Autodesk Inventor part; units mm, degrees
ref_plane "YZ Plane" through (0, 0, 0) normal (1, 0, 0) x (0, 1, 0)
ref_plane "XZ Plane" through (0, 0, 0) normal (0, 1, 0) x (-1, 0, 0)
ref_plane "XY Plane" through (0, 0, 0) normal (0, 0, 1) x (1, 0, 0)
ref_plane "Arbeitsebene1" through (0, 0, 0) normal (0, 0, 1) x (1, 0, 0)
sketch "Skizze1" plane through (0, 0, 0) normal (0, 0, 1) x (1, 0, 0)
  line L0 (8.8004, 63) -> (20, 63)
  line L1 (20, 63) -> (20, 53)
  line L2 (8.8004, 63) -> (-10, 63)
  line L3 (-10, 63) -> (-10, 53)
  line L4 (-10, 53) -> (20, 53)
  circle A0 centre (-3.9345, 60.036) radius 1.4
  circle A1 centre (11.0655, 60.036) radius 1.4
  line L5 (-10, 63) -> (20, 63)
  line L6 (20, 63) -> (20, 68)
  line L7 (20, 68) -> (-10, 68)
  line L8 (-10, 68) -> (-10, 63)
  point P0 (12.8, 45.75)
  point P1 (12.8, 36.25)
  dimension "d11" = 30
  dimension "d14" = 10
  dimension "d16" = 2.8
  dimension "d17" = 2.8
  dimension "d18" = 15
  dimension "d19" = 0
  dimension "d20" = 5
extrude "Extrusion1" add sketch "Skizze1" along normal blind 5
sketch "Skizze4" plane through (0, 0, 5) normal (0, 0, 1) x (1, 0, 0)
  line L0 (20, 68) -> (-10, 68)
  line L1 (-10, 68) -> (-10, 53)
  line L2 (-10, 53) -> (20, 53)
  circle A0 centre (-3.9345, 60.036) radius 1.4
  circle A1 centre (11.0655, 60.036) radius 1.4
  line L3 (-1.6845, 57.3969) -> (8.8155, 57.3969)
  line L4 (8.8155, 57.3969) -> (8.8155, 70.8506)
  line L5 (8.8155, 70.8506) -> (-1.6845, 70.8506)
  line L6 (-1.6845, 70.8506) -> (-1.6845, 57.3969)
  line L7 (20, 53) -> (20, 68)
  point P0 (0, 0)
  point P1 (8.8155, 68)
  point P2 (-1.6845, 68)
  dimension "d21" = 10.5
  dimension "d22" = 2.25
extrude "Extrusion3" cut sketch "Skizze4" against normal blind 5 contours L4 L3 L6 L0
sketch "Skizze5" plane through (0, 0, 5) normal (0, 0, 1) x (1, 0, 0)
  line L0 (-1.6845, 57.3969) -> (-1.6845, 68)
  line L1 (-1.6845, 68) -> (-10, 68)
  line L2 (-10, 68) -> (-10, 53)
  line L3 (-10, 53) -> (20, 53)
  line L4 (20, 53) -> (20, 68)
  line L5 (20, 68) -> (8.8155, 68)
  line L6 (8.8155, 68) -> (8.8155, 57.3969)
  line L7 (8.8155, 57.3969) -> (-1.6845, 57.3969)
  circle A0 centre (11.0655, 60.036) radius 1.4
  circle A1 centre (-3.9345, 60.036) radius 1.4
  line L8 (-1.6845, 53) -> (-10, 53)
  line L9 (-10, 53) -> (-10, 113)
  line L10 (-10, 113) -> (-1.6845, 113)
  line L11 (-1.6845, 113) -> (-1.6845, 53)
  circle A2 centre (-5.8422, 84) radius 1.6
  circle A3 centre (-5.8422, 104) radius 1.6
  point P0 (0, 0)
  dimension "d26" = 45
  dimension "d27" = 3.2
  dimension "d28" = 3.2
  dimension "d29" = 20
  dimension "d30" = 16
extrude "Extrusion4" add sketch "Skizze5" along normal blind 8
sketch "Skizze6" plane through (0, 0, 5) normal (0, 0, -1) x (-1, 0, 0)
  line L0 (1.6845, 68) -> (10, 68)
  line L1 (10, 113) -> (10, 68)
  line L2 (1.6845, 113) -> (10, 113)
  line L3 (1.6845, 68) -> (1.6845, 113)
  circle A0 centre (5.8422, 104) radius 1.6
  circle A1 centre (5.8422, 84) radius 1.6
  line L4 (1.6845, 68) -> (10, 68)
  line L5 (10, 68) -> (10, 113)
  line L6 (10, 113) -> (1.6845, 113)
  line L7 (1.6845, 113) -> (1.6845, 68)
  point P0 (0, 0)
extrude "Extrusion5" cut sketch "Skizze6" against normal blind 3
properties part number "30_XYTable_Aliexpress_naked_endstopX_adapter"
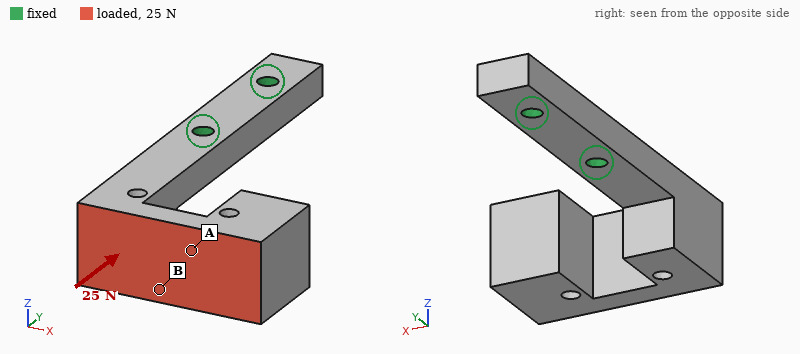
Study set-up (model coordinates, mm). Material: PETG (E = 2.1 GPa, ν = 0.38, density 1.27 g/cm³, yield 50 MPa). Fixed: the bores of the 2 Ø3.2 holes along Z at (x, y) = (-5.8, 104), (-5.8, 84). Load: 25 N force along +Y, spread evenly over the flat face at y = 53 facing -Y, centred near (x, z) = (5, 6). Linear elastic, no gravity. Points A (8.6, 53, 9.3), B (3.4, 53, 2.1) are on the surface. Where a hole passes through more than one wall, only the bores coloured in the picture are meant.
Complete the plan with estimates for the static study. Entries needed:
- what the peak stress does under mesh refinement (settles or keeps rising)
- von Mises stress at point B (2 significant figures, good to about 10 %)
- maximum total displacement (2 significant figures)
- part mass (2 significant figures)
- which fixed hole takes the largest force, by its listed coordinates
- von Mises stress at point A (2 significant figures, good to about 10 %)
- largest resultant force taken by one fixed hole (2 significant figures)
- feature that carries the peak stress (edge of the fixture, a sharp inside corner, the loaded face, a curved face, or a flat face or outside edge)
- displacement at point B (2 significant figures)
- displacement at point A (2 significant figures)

keeps rising
2.7 MPa
0.73 mm
7.7 g
(-5.8, 84)
1.2 MPa
25 N
edge of the fixture
0.43 mm
0.46 mm
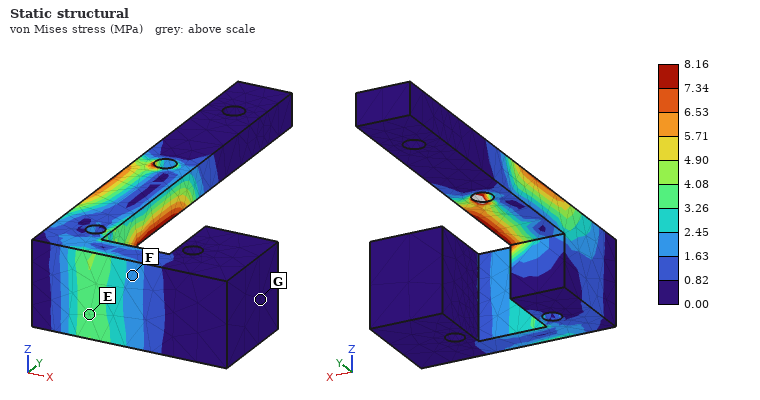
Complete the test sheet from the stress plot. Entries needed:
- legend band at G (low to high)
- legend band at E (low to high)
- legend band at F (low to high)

0.00 to 0.82 MPa
3.26 to 4.08 MPa
1.63 to 2.45 MPa
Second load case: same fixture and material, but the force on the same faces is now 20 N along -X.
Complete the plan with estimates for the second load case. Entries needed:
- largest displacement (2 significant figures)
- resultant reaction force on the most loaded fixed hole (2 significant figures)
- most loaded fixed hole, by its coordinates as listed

0.80 mm
31 N
(-5.8, 84)
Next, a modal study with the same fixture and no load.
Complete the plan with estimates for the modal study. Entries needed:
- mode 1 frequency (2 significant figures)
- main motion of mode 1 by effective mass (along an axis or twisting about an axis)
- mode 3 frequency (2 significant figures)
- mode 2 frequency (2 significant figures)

310 Hz
along Z
710 Hz
420 Hz
